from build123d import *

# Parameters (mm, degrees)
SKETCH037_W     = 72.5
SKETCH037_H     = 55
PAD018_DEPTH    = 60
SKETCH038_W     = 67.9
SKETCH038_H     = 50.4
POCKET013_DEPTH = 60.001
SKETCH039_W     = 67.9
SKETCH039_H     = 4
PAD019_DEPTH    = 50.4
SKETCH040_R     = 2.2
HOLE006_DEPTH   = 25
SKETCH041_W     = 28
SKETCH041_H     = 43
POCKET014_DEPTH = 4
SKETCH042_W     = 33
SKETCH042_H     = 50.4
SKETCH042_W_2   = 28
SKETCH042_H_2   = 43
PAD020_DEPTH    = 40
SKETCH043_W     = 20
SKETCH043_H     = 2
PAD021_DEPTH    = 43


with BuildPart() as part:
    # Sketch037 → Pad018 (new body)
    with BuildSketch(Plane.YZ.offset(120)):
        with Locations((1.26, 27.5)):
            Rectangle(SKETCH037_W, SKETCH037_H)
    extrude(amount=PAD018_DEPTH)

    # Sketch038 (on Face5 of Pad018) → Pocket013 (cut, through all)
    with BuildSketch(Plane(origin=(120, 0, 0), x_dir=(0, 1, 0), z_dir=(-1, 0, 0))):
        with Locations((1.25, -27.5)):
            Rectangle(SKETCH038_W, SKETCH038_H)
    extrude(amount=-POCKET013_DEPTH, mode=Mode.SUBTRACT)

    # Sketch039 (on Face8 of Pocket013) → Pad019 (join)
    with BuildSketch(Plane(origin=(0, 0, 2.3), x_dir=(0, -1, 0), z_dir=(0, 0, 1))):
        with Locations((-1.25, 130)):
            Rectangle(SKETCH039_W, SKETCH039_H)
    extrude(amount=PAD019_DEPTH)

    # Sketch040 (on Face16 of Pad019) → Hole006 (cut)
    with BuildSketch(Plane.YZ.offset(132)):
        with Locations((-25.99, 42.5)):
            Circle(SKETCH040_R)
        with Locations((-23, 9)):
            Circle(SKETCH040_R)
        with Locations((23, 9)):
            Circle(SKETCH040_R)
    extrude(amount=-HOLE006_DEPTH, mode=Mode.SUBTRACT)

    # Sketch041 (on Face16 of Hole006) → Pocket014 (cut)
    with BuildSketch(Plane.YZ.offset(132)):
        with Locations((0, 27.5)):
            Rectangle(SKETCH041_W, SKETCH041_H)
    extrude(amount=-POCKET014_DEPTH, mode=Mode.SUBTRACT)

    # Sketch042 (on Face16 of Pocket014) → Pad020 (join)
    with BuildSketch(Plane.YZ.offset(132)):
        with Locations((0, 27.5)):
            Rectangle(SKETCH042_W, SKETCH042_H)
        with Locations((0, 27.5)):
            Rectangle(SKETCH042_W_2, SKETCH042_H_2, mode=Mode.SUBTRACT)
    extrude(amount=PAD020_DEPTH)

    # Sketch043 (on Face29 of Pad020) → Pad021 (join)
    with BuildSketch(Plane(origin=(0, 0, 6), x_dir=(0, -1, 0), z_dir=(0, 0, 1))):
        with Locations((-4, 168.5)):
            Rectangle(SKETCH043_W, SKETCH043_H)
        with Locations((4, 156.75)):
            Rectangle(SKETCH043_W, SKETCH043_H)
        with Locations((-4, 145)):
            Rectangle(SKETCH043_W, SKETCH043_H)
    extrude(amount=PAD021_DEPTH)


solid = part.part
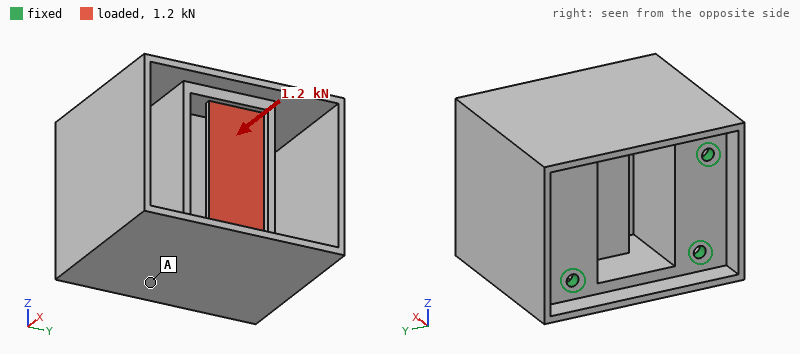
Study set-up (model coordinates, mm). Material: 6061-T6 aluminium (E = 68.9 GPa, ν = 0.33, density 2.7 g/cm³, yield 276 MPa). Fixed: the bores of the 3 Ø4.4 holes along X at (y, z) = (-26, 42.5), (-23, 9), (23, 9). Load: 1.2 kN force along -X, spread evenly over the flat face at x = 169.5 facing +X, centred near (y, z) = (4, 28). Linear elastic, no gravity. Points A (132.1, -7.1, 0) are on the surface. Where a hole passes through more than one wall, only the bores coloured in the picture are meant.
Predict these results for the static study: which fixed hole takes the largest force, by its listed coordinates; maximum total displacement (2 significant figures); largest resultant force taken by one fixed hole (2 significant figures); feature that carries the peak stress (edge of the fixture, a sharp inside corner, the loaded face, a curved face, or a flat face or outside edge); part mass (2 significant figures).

(23, 9)
0.22 mm
760 N
a flat face or outside edge
180 g
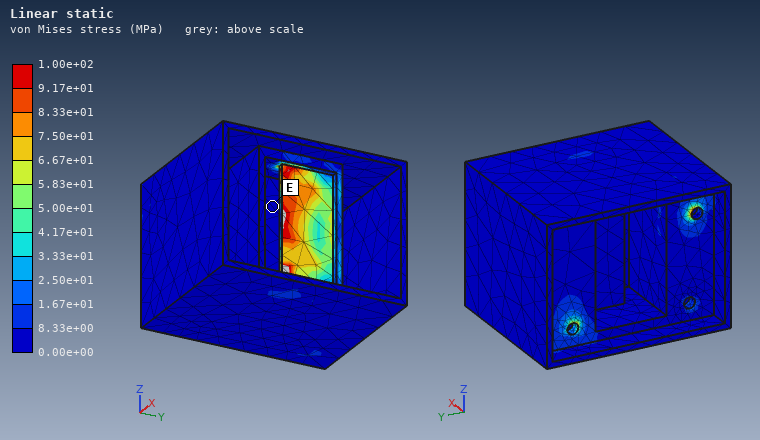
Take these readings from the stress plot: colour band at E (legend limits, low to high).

0.00e+00 to 8.33e+00 MPa
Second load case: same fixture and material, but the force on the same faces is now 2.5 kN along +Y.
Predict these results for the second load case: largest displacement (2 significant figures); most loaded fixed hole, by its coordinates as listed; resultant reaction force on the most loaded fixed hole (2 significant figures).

0.13 mm
(23, 9)
2.4 kN
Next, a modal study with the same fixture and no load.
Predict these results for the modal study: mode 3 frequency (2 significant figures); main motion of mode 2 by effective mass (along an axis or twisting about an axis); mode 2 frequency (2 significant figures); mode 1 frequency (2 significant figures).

4000 Hz
along Y
3800 Hz
2100 Hz
